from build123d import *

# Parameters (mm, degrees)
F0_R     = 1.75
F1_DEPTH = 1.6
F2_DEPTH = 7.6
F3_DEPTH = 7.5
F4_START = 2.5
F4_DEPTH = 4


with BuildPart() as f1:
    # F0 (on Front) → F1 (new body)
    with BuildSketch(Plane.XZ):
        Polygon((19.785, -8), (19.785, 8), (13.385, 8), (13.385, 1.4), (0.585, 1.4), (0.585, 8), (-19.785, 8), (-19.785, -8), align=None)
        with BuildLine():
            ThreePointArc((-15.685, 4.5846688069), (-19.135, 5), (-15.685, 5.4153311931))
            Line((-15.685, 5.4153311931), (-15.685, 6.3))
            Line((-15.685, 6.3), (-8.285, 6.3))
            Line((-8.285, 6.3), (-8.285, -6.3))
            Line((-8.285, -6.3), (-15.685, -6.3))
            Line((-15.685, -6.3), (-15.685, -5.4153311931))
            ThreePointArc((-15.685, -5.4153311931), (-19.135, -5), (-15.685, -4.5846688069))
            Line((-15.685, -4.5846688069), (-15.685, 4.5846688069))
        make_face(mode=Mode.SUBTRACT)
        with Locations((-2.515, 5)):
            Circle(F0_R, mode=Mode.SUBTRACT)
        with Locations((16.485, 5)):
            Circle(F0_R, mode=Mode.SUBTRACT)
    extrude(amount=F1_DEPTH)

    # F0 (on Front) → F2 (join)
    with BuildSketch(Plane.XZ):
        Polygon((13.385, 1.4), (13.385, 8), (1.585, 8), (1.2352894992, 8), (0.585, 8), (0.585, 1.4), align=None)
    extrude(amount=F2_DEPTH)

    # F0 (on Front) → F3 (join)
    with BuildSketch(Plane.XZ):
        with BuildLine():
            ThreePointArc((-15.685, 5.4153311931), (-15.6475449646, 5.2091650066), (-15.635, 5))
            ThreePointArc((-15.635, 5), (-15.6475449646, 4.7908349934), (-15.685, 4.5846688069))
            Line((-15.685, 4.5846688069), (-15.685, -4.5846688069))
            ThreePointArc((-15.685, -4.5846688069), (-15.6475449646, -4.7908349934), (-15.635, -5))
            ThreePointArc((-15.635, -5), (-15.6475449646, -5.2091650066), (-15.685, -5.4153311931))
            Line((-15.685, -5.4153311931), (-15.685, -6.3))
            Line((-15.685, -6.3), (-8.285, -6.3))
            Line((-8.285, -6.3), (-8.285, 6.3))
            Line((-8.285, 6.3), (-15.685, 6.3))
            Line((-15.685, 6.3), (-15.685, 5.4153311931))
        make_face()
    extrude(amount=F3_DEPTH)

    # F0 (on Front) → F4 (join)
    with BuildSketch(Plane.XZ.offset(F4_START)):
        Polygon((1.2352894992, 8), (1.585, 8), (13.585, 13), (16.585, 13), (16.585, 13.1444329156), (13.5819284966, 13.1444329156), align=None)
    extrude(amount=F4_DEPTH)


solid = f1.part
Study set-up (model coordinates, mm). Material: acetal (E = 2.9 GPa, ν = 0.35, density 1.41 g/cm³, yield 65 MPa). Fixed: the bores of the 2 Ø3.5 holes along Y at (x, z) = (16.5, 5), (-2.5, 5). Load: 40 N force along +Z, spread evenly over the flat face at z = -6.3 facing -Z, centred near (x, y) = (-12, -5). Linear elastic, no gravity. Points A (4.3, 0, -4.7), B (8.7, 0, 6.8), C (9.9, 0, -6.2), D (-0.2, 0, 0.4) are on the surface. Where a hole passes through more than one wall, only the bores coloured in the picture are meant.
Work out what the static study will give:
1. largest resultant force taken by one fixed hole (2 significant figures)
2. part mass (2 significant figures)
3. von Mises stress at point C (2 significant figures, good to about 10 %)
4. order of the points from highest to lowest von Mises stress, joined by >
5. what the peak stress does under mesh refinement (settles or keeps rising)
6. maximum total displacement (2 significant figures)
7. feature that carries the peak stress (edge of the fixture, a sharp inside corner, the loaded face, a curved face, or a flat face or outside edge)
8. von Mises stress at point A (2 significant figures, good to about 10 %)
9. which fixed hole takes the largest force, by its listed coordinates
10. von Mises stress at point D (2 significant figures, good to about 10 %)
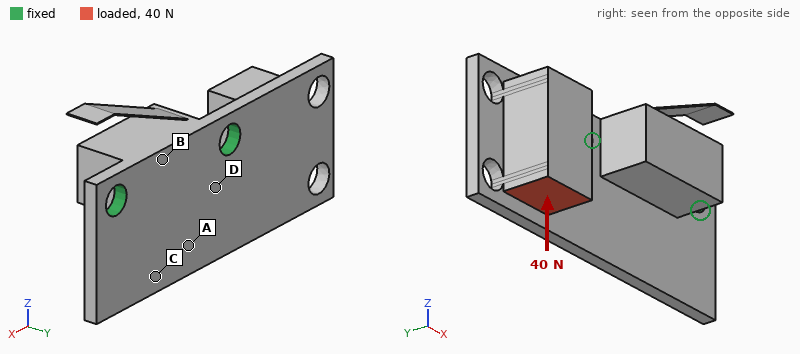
55 N
2.8 g
3.6 MPa
D > A > C > B
keeps rising
0.47 mm
edge of the fixture
7.0 MPa
(-2.5, 5)
10 MPa
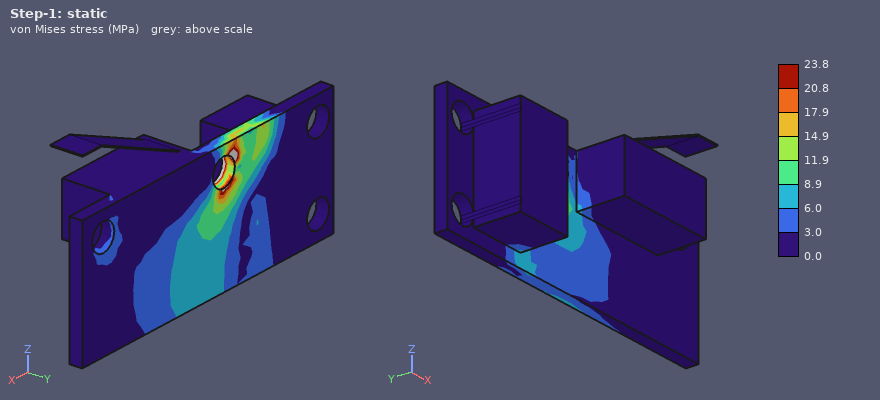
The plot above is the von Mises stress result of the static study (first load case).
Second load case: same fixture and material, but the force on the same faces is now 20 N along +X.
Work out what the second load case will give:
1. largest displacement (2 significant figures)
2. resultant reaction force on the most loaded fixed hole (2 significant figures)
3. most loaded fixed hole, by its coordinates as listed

0.47 mm
15 N
(16.5, 5)
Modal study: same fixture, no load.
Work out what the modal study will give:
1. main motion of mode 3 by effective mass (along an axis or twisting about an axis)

along Y
